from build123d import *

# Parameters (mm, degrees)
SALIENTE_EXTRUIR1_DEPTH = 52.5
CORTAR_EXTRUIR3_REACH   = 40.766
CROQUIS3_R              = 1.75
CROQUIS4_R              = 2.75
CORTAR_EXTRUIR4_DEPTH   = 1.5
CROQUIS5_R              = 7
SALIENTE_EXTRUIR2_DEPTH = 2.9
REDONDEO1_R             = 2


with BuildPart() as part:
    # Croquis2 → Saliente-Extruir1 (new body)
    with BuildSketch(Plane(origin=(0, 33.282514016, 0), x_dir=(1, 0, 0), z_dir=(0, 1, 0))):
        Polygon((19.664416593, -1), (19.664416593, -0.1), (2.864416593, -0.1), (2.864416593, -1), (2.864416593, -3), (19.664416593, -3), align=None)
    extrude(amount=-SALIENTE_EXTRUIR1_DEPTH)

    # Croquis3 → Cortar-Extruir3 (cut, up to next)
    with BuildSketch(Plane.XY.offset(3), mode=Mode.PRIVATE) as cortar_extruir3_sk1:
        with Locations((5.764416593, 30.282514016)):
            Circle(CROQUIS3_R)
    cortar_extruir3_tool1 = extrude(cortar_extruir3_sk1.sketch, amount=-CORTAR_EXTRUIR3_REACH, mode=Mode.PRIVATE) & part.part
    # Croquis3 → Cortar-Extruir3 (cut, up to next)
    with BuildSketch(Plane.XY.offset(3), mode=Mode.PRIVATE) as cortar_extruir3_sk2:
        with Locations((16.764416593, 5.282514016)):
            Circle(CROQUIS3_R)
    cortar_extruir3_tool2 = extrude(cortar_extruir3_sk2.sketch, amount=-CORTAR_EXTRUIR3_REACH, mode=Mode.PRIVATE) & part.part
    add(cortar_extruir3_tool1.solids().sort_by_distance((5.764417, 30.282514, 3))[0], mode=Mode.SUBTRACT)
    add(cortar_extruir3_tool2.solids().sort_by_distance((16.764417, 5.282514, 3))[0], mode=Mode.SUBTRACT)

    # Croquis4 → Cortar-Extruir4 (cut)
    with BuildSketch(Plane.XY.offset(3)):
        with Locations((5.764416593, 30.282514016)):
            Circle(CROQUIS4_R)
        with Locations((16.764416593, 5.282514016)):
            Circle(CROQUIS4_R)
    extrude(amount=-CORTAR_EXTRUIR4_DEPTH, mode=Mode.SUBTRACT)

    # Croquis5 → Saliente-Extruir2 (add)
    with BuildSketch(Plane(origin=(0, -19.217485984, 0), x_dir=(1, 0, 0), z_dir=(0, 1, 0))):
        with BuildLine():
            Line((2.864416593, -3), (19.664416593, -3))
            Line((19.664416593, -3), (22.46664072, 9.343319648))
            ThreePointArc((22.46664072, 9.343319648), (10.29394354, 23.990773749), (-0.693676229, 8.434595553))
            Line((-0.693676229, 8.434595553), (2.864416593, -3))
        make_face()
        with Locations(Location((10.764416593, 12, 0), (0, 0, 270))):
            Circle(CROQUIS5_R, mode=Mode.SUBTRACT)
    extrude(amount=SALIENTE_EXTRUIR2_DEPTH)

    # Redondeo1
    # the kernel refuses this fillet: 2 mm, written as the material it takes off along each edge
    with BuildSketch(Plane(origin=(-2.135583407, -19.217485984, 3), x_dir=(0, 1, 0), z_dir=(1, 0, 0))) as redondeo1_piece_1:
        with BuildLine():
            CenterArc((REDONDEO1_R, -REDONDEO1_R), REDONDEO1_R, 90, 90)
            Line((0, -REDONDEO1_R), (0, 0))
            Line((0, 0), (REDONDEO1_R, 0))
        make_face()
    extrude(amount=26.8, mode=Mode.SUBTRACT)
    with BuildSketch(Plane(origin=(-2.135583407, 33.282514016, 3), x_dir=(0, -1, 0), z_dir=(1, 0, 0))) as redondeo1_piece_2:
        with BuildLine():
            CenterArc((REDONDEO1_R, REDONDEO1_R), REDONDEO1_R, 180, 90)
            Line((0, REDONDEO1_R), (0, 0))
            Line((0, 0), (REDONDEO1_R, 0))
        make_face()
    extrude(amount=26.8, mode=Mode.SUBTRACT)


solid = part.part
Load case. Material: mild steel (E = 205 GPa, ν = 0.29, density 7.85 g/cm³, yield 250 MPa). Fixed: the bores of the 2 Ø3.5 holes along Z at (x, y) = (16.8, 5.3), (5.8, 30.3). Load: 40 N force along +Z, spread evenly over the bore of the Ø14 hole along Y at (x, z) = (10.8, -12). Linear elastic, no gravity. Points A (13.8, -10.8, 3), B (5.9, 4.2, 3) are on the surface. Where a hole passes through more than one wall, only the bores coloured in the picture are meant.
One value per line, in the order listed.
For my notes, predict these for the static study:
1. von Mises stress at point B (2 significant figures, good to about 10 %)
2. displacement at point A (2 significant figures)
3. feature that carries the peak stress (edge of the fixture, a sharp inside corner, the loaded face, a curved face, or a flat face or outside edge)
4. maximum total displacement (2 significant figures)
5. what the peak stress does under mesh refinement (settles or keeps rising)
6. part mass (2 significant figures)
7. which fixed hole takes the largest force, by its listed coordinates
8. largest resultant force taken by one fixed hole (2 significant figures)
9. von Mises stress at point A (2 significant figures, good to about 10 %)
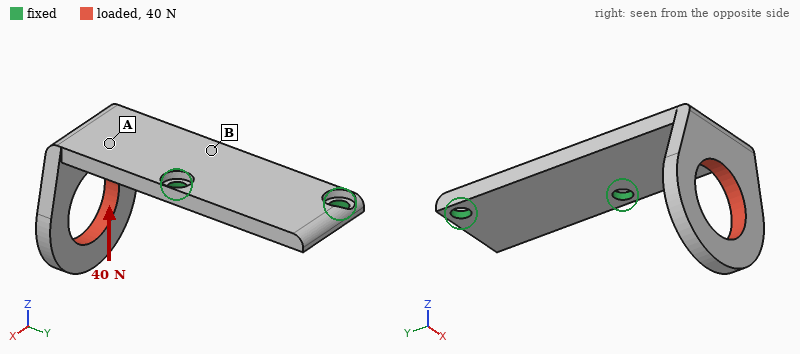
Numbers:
28 MPa
23 µm
edge of the fixture
68 µm
keeps rising
27 g
(16.8, 5.3)
74 N
11 MPa
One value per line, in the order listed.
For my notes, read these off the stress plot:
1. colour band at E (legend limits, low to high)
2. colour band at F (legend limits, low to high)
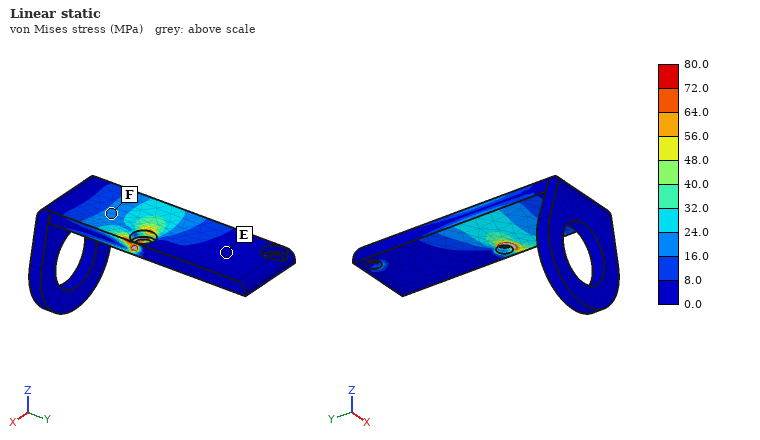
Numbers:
0.0 to 8.0 MPa
16.0 to 24.0 MPa
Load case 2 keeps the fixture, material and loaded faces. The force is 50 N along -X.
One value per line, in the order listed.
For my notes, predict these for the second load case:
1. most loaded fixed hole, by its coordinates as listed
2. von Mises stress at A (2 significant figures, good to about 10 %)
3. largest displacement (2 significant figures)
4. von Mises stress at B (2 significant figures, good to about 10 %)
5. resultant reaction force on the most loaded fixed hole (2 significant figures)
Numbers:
(16.8, 5.3)
23 MPa
54 µm
19 MPa
85 N
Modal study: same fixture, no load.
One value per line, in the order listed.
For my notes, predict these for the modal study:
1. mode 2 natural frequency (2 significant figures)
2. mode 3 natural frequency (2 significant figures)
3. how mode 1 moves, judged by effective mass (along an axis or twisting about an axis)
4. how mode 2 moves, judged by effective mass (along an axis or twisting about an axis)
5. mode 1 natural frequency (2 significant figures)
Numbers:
2000 Hz
3500 Hz
along Z
along X
1300 Hz
